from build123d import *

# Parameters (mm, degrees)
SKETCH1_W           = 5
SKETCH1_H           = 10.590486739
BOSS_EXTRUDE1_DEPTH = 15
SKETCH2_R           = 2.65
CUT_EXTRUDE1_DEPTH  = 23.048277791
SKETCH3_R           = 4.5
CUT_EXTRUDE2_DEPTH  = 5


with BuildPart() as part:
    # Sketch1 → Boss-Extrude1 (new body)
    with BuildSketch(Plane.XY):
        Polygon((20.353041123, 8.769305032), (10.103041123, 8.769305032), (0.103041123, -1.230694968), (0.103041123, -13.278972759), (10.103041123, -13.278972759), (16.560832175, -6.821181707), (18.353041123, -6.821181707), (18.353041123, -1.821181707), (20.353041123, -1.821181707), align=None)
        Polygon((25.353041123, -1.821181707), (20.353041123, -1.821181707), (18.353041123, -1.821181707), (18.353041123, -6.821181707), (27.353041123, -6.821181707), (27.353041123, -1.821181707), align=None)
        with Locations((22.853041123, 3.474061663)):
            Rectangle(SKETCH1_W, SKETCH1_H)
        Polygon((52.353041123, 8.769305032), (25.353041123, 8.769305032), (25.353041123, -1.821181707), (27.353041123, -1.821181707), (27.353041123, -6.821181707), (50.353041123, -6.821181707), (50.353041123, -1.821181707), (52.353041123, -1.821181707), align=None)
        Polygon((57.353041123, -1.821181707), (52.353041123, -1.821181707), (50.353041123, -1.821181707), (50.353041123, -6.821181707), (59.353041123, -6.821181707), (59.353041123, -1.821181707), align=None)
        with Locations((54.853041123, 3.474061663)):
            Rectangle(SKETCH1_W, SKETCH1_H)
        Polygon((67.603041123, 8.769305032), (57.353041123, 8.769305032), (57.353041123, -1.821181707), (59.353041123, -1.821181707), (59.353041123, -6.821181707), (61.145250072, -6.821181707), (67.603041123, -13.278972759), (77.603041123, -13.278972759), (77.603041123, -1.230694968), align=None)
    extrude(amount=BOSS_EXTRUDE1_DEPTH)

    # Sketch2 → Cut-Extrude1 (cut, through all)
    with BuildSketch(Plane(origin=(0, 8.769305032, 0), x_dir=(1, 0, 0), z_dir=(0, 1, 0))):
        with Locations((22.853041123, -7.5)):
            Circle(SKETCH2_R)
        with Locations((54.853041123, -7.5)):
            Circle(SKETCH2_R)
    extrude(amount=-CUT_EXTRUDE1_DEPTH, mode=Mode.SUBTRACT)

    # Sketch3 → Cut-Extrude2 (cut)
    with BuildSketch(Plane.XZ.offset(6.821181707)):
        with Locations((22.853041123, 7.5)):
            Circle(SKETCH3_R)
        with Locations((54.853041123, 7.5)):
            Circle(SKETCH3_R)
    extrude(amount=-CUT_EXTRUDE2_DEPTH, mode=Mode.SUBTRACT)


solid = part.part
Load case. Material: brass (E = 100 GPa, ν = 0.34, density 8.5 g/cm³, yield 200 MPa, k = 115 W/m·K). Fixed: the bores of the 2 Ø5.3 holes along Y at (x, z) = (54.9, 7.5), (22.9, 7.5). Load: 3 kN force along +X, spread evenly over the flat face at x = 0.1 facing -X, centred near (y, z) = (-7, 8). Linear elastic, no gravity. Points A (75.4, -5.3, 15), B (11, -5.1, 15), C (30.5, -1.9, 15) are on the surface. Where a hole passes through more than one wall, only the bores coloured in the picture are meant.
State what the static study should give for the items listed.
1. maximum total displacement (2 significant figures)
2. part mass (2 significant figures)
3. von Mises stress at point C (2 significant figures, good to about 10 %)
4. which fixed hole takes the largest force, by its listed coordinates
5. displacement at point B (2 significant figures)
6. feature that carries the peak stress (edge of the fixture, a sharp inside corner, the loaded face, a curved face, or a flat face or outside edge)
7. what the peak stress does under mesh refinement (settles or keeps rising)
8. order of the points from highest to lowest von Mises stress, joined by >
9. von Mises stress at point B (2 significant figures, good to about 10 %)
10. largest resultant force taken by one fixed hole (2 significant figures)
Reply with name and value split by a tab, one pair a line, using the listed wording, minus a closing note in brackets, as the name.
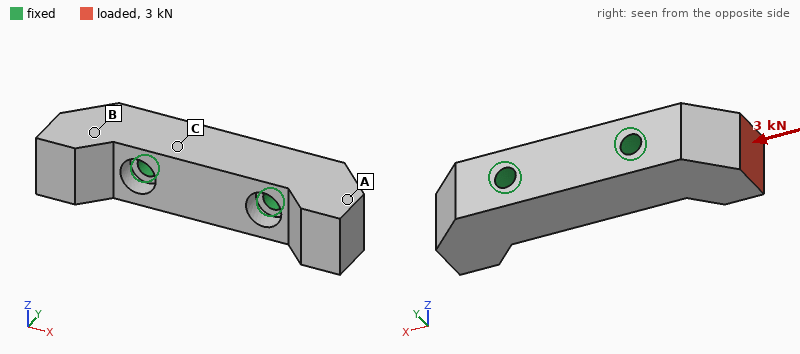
maximum total displacement	31 µm
part mass	150 g
von Mises stress at point C	19 MPa
which fixed hole takes the largest force, by its listed coordinates	(22.9, 7.5)
displacement at point B	13 µm
feature that carries the peak stress	edge of the fixture
what the peak stress does under mesh refinement	keeps rising
order of the points from highest to lowest von Mises stress, joined by >	B > C > A
von Mises stress at point B	32 MPa
largest resultant force taken by one fixed hole	2.4 kN
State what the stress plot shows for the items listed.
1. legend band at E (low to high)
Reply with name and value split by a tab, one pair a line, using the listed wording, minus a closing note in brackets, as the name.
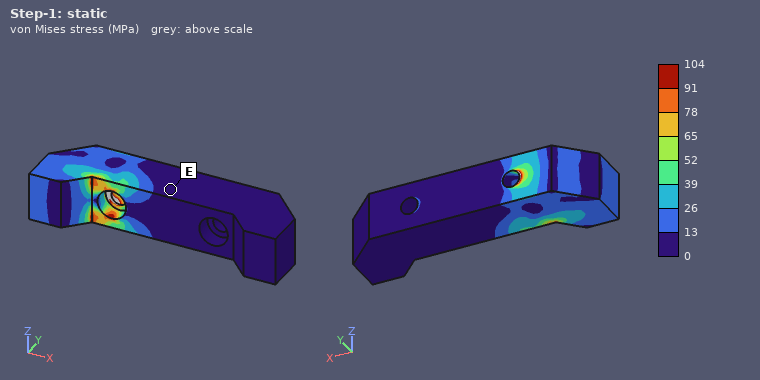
legend band at E	0 to 13 MPa
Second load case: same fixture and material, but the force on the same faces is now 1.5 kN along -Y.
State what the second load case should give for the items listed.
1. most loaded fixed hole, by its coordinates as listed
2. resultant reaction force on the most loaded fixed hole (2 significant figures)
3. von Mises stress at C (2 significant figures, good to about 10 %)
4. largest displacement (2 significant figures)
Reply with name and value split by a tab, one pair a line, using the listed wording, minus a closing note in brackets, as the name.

most loaded fixed hole, by its coordinates as listed	(22.9, 7.5)
resultant reaction force on the most loaded fixed hole	1.9 kN
von Mises stress at C	15 MPa
largest displacement	33 µm
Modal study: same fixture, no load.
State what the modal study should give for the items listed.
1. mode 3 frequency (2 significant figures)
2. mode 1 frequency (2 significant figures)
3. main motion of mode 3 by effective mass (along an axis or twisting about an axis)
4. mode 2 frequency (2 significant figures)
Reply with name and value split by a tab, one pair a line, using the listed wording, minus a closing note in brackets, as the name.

mode 3 frequency	9100 Hz
mode 1 frequency	8400 Hz
main motion of mode 3 by effective mass	along Y
mode 2 frequency	8600 Hz
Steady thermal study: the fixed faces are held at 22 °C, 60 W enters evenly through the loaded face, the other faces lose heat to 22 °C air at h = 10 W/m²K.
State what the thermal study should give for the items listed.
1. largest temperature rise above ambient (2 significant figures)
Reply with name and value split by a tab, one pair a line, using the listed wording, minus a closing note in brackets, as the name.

largest temperature rise above ambient	63 K
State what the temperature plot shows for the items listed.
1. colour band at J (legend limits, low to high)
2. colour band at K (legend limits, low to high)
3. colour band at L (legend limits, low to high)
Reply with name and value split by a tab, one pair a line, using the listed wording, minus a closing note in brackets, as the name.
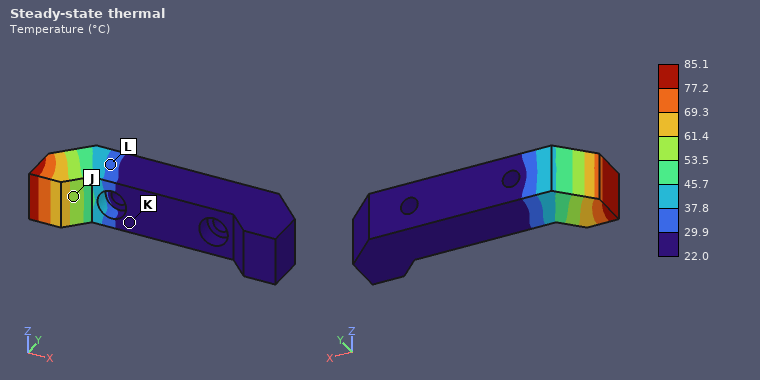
colour band at J	53.5 to 61.4 °C
colour band at K	22.0 to 29.9 °C
colour band at L	29.9 to 37.8 °C
